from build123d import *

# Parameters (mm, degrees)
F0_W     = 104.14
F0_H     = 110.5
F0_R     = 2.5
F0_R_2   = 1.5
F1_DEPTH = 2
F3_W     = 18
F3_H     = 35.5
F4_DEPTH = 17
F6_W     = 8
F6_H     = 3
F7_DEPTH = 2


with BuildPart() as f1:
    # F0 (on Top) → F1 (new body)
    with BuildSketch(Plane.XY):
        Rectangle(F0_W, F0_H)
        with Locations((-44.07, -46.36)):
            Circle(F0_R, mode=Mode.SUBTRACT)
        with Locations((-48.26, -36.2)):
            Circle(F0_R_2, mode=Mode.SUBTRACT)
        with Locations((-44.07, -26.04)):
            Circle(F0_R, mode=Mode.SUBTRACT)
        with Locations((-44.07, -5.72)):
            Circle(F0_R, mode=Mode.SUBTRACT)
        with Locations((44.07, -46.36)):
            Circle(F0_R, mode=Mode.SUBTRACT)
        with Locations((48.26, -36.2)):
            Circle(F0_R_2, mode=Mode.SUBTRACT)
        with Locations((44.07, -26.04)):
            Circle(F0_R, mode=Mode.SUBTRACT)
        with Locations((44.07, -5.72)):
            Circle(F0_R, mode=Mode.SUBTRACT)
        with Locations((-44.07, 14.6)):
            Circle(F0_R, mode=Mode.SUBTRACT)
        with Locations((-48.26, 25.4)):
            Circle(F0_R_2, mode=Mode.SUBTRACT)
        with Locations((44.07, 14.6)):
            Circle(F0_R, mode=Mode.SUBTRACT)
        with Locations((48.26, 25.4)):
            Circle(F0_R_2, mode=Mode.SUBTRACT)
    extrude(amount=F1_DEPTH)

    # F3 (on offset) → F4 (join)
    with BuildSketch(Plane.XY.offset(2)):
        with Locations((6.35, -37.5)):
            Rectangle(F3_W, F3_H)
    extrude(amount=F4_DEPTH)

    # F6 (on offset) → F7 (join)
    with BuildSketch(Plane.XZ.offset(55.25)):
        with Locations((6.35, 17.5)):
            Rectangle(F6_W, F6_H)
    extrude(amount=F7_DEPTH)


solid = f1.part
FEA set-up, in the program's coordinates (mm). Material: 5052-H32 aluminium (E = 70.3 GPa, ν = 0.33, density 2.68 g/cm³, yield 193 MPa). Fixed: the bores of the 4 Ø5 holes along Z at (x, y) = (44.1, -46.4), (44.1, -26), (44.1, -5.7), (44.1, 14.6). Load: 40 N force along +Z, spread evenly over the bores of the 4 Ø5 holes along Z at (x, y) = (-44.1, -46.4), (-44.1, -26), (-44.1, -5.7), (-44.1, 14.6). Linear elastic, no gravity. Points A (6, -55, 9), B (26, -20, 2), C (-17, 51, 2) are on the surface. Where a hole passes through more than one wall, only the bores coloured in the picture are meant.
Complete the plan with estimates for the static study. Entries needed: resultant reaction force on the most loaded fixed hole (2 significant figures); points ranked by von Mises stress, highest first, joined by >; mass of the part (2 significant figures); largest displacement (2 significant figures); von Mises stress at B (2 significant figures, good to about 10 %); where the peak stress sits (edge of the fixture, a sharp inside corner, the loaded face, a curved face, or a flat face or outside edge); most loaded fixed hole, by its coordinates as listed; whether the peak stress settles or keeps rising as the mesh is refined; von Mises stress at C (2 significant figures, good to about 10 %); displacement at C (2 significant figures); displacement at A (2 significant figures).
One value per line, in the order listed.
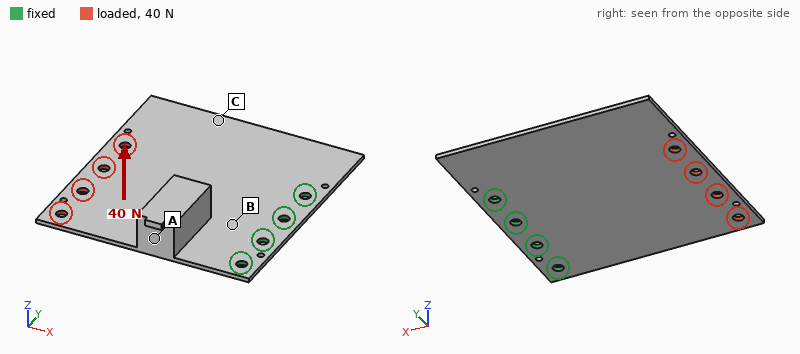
17 N
B > C > A
90 g
1.9 mm
43 MPa
edge of the fixture
(44.1, -5.7)
keeps rising
11 MPa
0.76 mm
0.47 mm
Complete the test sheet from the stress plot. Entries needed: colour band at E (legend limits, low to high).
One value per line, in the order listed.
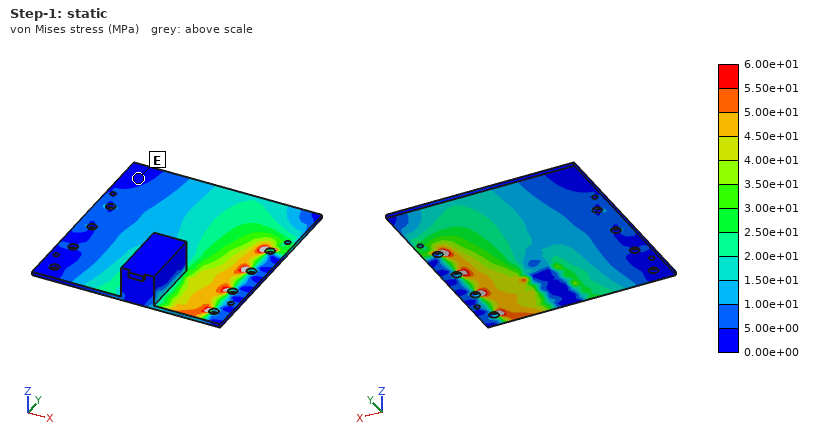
0.00e+00 to 5.00e+00 MPa
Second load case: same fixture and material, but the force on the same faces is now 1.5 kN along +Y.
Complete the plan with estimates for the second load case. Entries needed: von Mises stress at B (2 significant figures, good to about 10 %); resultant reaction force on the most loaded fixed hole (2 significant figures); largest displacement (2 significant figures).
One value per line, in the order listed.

27 MPa
2.0 kN
0.11 mm
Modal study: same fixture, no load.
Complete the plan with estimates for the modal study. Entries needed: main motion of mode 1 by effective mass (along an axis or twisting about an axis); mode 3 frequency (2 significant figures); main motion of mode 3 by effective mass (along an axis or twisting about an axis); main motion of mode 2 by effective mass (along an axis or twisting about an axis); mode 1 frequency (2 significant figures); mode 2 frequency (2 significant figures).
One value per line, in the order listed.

along Z
810 Hz
along Z
twisting about X
180 Hz
370 Hz
